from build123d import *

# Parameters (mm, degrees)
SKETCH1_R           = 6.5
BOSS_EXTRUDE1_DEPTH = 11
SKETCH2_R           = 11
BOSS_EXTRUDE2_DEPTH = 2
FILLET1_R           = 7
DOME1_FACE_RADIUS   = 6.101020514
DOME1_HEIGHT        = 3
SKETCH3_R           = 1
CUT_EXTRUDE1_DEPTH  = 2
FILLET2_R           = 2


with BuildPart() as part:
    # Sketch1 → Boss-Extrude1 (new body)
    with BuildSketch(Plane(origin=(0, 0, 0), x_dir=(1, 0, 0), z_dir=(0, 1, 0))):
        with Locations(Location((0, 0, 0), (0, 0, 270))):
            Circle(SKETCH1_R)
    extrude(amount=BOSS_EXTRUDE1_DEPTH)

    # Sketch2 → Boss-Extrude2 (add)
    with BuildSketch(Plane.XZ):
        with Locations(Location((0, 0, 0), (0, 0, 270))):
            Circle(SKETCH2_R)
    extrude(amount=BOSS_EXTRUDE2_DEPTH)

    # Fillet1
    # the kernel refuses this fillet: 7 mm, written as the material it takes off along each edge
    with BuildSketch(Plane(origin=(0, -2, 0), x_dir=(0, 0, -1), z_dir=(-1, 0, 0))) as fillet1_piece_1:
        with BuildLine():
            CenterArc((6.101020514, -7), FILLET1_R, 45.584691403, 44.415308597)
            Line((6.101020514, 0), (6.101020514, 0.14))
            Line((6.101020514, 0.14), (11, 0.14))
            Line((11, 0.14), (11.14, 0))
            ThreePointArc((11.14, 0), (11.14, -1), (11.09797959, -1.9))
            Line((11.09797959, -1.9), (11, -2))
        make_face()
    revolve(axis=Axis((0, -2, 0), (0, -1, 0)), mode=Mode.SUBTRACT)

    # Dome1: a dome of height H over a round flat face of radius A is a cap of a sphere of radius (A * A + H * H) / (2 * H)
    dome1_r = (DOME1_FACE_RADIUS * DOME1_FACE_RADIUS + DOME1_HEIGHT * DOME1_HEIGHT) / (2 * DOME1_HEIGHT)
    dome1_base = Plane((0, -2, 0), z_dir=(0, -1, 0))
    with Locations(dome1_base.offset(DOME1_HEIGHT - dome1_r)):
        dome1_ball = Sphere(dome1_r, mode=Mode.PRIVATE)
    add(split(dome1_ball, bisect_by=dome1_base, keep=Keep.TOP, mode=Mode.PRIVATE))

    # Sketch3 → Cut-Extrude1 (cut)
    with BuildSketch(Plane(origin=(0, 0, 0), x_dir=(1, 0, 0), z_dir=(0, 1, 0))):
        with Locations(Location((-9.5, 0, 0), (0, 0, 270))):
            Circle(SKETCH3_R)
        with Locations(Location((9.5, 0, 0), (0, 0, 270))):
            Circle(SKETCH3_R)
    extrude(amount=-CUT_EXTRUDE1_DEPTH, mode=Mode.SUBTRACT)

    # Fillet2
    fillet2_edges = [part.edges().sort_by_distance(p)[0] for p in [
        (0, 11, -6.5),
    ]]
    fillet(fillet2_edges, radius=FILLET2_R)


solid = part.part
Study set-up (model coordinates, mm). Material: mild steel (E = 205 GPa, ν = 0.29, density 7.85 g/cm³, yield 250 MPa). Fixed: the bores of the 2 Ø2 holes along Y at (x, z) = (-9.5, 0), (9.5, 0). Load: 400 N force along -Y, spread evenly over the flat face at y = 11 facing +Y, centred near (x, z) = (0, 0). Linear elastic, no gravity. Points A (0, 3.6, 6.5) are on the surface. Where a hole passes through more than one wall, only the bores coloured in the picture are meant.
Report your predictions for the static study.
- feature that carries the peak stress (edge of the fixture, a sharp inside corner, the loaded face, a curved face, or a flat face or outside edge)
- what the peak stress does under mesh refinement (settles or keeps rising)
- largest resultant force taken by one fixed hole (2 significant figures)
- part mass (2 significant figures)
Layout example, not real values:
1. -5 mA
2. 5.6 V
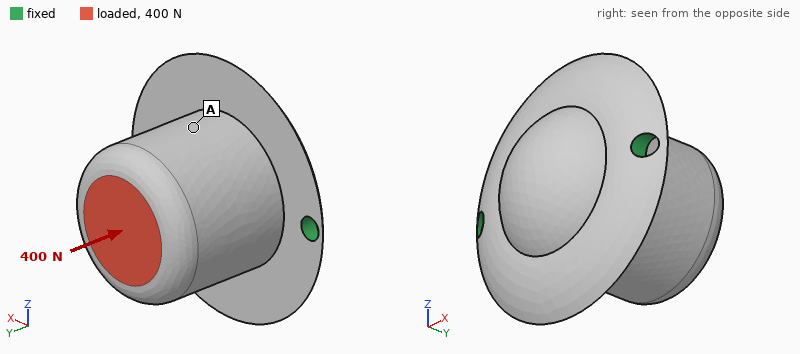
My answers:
1. edge of the fixture
2. keeps rising
3. 200 N
4. 17 g
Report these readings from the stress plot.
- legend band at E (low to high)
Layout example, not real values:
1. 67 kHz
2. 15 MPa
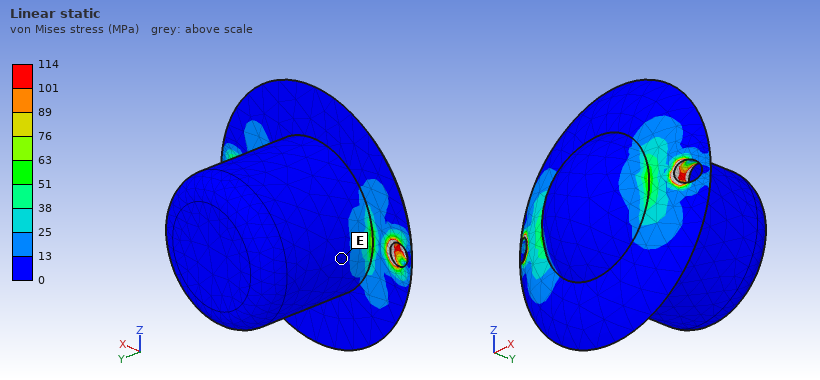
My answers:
1. 0 to 13 MPa
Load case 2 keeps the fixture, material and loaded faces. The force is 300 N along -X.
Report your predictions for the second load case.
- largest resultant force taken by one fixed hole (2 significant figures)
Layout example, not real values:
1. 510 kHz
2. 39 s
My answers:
1. 270 N
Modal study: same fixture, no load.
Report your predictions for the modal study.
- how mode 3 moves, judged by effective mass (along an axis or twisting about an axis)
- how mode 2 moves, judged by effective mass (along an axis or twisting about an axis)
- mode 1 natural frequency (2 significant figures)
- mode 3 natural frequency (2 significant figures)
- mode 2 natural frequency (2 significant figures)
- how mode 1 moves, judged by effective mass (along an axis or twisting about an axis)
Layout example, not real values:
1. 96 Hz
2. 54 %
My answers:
1. along X
2. along Y
3. 4300 Hz
4. 17 kHz
5. 16 kHz
6. along Z
